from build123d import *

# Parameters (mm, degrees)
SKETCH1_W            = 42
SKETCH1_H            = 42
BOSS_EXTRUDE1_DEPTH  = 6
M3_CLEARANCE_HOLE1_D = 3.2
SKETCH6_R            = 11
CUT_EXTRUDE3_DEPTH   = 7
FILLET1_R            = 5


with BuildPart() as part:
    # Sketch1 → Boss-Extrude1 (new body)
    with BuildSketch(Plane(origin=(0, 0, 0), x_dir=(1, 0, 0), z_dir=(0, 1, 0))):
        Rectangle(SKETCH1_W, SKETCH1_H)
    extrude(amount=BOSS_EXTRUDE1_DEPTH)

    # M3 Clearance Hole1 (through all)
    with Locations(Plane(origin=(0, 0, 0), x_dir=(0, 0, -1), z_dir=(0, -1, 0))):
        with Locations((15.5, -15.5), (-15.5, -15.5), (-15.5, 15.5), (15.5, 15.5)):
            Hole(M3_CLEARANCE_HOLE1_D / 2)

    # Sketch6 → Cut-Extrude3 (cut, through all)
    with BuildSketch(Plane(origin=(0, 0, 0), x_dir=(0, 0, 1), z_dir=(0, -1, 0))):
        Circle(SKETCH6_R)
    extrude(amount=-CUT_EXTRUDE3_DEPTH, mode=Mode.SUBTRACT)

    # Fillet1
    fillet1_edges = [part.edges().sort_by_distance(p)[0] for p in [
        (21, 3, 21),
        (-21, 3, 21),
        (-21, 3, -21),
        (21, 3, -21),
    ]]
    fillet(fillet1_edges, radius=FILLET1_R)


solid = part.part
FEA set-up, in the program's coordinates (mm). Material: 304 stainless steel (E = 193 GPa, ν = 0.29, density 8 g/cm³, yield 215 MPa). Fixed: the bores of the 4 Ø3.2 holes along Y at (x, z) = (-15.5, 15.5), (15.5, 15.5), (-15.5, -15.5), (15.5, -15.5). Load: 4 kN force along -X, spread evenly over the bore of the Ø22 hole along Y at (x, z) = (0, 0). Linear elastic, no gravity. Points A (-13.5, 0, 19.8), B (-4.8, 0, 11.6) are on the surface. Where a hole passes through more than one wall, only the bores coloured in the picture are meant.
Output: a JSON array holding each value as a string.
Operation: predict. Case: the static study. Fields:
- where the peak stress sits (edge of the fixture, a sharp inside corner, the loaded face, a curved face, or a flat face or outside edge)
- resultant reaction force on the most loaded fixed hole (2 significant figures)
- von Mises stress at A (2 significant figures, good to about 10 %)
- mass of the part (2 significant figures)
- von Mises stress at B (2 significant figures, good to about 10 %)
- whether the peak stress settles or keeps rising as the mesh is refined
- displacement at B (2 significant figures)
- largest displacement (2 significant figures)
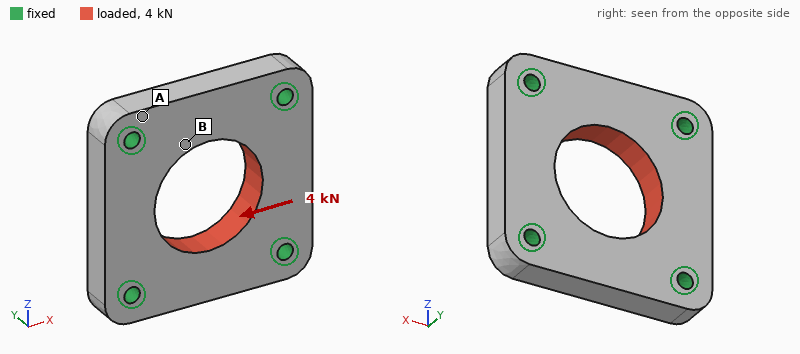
["edge of the fixture", "1.0 kN", "6.2 MPa", "64 g", "18 MPa", "keeps rising", "0.92 µm", "2.2 µm"]
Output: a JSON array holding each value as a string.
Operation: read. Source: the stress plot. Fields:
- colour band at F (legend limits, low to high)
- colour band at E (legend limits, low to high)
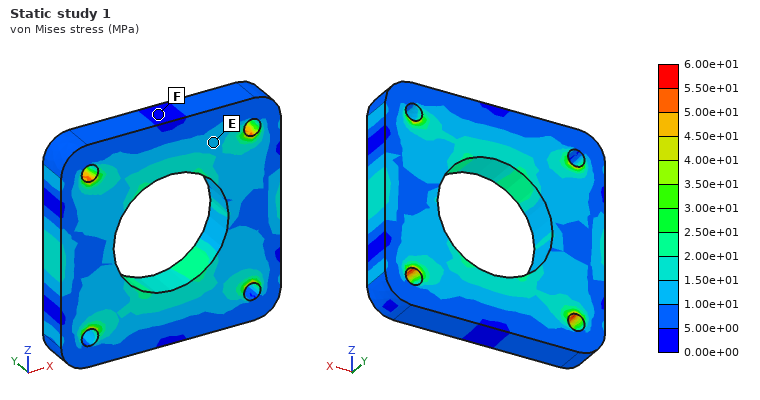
["0.00e+00 to 5.00e+00 MPa", "1.00e+01 to 1.50e+01 MPa"]
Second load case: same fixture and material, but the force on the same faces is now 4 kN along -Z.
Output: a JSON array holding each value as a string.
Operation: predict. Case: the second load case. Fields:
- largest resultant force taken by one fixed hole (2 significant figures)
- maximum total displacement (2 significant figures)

["1.0 kN", "2.2 µm"]
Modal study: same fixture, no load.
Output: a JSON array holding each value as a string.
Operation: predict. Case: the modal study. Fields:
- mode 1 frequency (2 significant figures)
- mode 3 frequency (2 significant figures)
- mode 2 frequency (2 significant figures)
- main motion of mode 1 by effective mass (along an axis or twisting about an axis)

["25 kHz", "27 kHz", "27 kHz", "along Y"]
